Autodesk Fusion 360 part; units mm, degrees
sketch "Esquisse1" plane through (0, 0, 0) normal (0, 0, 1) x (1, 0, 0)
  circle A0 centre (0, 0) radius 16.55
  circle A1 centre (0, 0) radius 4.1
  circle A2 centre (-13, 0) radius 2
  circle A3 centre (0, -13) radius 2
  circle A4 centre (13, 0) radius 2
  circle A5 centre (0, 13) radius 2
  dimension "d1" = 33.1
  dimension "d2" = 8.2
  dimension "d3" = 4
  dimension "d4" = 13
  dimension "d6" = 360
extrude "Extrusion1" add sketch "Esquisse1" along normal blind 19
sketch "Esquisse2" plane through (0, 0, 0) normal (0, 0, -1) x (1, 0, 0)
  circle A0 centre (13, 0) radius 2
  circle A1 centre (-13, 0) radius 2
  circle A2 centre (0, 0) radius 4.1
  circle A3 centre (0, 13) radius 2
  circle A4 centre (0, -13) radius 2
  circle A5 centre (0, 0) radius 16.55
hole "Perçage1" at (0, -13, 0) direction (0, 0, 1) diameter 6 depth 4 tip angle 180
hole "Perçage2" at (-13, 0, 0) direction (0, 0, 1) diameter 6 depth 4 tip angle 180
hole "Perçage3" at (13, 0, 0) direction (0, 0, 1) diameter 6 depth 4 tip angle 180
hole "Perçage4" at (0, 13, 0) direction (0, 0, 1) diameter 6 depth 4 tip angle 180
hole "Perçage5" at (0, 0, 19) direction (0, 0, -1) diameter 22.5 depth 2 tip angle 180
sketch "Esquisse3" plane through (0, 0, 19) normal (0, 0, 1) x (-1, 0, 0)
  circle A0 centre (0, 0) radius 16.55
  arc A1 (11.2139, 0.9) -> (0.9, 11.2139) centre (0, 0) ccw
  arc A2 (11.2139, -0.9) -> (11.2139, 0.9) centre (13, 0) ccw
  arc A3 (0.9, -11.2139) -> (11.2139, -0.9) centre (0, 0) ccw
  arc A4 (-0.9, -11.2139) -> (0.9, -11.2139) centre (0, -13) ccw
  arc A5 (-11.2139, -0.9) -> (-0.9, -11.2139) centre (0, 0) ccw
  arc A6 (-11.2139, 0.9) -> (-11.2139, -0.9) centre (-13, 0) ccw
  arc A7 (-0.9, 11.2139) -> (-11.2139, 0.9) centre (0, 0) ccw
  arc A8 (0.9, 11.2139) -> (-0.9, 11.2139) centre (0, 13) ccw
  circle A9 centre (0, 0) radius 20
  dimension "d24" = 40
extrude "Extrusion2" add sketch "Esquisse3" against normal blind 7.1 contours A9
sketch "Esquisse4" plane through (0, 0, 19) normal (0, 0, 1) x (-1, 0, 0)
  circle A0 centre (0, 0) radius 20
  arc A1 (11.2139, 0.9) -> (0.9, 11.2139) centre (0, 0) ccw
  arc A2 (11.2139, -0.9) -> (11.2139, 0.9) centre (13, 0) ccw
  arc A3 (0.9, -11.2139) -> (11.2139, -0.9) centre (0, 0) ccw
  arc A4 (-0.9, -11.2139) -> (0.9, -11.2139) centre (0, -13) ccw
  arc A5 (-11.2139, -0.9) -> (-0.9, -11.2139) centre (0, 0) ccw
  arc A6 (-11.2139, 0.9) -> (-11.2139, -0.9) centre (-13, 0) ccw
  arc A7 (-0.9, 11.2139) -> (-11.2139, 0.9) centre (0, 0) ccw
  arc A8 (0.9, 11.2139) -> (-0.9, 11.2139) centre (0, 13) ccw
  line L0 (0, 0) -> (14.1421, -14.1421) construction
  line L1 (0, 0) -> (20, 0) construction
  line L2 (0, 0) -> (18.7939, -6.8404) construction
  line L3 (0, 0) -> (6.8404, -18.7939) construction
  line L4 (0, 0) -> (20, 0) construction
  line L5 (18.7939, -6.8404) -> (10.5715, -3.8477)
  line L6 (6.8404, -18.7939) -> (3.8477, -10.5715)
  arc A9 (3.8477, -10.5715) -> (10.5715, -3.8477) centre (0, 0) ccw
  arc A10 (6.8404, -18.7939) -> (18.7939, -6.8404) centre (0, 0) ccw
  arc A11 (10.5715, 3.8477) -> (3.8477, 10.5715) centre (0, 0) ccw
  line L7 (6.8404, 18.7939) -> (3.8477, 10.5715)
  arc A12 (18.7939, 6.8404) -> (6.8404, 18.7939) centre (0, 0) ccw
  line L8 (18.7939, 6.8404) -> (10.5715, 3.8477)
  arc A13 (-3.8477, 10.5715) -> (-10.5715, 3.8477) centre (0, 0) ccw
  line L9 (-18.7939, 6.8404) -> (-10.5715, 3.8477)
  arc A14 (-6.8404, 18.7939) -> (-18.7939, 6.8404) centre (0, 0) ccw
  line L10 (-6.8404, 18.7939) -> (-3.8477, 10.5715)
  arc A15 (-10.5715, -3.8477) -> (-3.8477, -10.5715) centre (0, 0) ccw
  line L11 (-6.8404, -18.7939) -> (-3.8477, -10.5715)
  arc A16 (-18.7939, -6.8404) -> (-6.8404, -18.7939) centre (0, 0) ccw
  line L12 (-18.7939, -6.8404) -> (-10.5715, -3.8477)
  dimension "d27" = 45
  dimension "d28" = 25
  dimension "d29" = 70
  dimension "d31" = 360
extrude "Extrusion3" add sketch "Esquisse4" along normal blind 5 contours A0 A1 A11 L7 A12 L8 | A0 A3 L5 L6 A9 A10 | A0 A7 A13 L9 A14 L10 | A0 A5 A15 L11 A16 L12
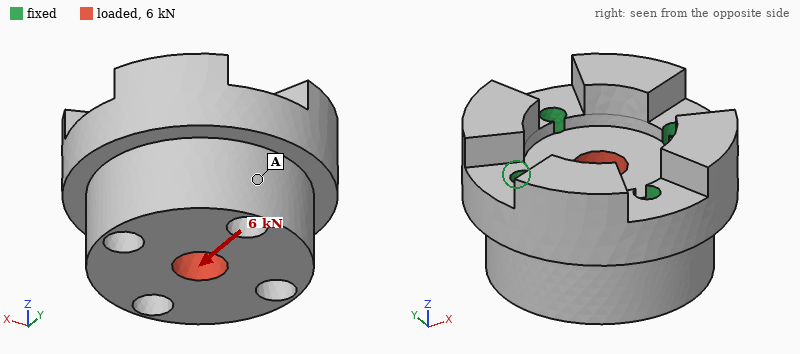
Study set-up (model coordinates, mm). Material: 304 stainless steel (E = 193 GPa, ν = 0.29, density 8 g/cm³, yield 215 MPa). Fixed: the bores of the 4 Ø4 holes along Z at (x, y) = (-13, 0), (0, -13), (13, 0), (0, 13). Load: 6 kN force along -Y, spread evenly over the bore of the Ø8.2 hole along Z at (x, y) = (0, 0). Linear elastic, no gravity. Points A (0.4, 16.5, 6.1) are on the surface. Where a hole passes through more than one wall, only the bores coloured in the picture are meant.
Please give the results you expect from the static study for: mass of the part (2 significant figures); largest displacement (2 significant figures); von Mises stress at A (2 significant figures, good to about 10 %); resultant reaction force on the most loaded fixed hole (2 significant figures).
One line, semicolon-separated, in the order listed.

150 g; 1.0 µm; 5.8 MPa; 1.9 kN
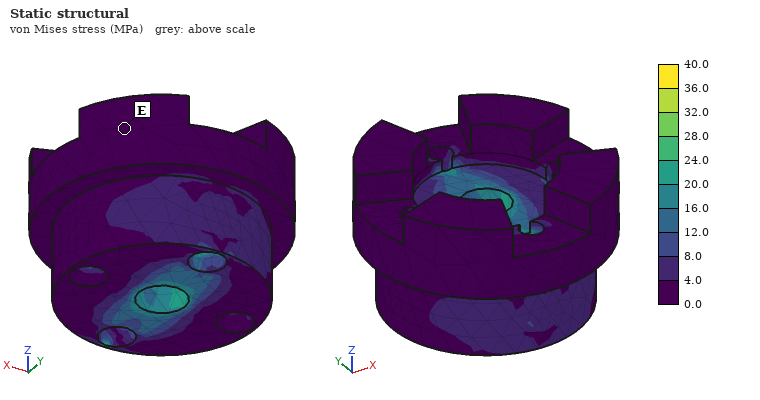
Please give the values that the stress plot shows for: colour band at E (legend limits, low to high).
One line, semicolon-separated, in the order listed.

0.0 to 4.0 MPa
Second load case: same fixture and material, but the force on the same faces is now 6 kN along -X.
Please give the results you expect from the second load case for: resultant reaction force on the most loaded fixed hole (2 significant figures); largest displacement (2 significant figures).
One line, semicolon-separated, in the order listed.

1.9 kN; 1.0 µm
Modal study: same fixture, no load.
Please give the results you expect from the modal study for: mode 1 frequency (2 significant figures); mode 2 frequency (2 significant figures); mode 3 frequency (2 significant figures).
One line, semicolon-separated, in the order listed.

36 kHz; 37 kHz; 37 kHz
